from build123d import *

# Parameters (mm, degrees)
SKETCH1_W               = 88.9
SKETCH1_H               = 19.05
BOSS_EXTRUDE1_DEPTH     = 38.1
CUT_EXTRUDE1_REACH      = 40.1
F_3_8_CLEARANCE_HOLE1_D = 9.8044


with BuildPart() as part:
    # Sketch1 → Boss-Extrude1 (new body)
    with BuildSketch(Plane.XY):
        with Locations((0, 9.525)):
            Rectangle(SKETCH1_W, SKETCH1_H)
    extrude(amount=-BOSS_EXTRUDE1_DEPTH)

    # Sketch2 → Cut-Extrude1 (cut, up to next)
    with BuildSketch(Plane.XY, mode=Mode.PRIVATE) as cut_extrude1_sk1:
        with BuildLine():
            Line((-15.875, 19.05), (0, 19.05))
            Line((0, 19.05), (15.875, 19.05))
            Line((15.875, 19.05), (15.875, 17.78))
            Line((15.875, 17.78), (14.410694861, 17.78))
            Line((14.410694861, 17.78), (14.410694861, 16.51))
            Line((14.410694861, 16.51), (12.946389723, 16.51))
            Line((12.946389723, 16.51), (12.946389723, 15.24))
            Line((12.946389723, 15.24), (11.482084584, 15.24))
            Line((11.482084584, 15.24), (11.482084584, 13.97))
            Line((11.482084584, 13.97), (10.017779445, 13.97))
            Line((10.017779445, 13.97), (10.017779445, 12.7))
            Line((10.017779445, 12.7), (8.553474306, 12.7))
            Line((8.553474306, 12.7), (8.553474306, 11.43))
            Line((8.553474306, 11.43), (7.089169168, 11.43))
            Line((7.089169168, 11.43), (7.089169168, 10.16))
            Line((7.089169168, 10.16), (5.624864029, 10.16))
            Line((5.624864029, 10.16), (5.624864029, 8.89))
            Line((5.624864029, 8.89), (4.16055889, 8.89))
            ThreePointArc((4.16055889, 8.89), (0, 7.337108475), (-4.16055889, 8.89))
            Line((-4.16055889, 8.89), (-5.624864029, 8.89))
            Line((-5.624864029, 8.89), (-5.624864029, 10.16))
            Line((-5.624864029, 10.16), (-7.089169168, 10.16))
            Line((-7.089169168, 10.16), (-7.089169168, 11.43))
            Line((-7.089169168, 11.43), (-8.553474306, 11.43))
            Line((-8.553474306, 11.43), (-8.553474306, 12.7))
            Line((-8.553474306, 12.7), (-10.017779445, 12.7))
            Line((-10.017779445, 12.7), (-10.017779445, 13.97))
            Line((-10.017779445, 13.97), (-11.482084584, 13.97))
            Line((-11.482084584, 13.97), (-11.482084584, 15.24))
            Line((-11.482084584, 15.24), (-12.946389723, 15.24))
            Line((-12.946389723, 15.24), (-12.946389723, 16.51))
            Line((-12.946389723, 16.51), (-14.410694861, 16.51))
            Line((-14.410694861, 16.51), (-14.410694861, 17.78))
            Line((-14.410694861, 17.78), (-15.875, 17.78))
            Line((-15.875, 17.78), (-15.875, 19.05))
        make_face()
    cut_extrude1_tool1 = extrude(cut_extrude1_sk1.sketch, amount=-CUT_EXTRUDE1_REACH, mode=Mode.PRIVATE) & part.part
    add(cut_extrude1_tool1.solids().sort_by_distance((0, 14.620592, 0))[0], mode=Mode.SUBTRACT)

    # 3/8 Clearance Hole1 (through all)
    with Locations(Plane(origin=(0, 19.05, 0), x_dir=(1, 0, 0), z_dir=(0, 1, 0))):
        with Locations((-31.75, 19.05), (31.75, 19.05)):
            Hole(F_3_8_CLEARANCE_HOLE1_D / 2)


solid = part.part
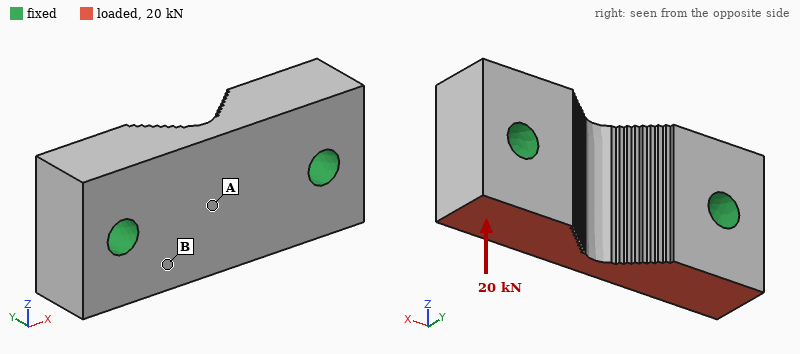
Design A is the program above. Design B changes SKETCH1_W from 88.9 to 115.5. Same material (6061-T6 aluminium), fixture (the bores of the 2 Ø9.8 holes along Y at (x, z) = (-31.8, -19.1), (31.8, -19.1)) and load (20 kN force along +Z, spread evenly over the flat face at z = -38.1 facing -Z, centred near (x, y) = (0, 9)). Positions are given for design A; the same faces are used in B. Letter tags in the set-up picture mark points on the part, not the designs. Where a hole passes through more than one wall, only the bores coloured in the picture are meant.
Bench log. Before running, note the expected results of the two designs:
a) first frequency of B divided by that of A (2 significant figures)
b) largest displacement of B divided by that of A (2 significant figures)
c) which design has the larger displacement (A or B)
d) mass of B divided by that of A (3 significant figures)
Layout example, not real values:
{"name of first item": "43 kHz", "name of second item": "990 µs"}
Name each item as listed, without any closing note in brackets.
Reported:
{"first frequency of B divided by that of A": "0.82", "largest displacement of B divided by that of A": "0.70", "which design has the larger displacement": "A", "mass of B divided by that of A": "1.36"}
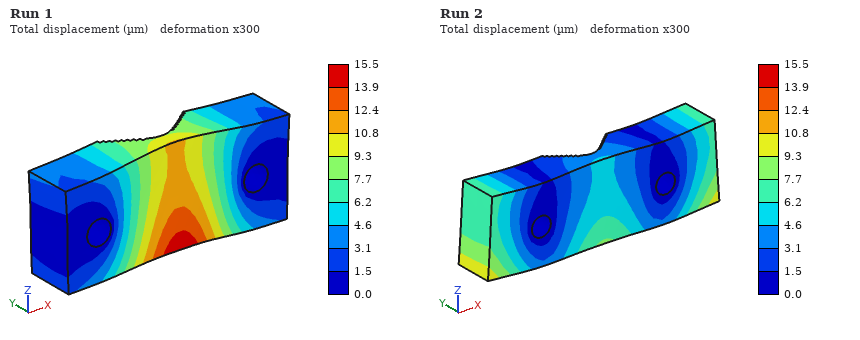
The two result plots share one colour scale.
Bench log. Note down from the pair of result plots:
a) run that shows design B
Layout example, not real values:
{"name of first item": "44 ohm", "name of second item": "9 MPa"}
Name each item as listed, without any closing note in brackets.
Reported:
{"run that shows design B": "Run 2"}
